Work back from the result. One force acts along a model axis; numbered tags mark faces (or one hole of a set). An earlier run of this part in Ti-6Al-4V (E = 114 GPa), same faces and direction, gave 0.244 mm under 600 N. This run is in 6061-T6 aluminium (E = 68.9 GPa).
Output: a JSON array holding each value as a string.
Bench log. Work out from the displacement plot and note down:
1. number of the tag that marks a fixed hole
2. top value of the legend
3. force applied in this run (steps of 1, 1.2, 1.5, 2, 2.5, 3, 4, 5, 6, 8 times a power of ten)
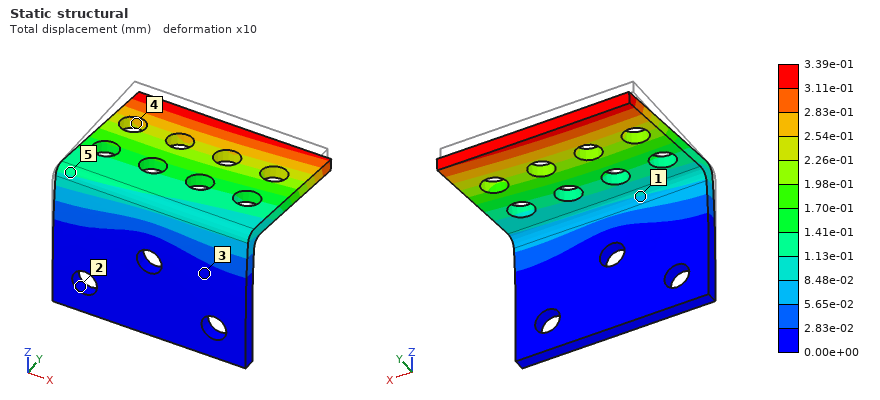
["2", "3.39e-01 mm", "500 N"]
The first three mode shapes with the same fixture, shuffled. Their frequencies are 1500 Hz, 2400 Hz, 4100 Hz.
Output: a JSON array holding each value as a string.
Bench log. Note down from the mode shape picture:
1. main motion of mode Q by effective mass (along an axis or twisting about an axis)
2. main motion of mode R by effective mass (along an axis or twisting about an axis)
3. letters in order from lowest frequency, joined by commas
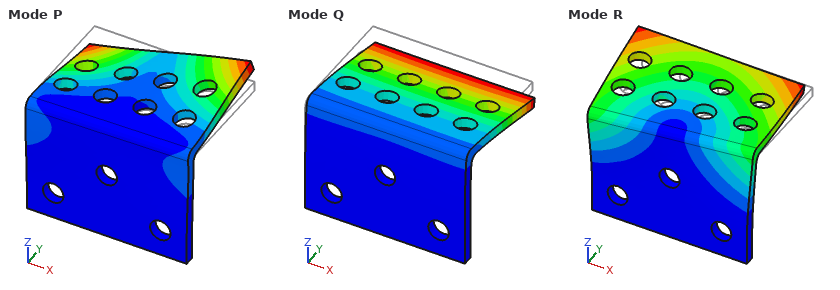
["along Z", "along X", "Q, R, P"]
